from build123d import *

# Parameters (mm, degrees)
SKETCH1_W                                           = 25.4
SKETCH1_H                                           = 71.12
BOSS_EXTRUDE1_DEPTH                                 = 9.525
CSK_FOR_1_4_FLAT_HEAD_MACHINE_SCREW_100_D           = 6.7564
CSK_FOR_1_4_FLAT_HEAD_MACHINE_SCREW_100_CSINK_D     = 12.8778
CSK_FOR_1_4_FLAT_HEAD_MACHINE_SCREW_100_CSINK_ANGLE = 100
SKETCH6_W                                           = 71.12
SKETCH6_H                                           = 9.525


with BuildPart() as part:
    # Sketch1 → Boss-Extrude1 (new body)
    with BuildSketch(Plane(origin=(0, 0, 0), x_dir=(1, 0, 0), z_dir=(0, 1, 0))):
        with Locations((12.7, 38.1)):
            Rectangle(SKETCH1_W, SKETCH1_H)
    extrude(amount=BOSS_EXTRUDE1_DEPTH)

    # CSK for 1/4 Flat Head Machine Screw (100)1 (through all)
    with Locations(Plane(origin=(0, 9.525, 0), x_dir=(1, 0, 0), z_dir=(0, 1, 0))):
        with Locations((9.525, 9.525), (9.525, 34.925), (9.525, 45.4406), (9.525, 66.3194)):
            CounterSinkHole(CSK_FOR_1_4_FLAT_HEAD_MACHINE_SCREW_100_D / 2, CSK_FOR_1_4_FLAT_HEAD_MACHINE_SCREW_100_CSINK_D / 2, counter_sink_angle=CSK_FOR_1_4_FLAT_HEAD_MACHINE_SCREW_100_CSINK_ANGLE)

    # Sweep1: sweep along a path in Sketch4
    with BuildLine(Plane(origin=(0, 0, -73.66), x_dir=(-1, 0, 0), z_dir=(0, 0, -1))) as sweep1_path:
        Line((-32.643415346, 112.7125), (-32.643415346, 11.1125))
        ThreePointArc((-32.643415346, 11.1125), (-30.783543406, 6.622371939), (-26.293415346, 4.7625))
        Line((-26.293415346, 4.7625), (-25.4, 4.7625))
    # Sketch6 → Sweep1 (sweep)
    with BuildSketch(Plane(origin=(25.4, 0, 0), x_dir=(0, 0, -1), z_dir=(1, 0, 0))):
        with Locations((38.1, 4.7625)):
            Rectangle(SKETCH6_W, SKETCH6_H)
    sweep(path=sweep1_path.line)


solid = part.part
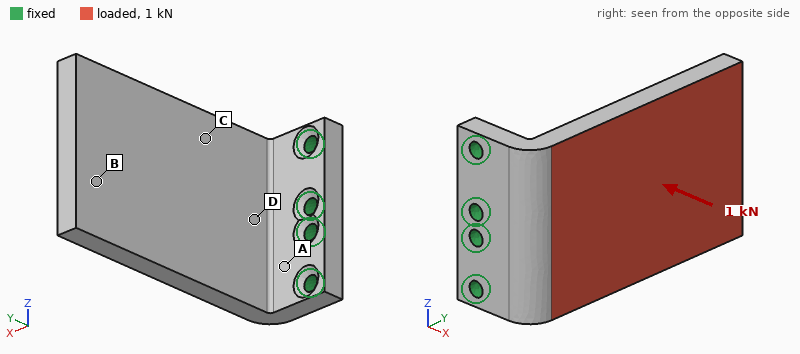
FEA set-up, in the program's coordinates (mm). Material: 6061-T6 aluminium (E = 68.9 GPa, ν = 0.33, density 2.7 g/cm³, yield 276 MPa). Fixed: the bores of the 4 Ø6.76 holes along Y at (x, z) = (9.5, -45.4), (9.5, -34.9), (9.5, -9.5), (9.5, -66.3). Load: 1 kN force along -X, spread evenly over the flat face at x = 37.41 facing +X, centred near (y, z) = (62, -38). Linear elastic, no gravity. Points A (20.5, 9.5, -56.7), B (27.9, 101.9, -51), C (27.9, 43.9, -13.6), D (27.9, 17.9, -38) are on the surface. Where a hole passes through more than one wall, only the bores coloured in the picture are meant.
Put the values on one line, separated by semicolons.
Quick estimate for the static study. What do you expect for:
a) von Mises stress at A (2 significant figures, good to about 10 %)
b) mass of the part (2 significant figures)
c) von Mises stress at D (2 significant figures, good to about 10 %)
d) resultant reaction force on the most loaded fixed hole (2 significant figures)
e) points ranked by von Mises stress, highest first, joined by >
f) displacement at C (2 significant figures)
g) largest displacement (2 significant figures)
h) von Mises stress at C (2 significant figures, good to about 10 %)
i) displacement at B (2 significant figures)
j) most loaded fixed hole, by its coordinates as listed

50 MPa; 250 g; 37 MPa; 440 N; A > D > C > B; 0.23 mm; 0.83 mm; 21 MPa; 0.72 mm; (9.5, -34.9)
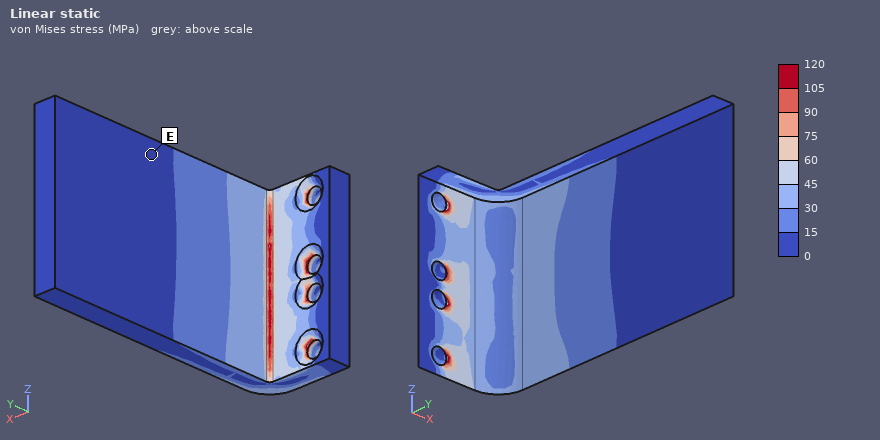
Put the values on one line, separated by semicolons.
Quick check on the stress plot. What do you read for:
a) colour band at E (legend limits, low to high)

0 to 15 MPa
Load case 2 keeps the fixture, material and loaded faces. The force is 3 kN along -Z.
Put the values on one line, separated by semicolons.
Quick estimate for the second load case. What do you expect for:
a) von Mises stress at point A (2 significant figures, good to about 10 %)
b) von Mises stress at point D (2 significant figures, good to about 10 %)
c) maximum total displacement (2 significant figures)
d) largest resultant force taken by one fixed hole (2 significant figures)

54 MPa; 25 MPa; 0.28 mm; 3.3 kN
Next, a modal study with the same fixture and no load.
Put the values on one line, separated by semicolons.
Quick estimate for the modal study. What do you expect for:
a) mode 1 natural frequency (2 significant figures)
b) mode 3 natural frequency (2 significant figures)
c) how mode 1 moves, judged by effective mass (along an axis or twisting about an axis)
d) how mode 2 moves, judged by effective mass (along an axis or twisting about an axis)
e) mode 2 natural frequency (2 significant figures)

500 Hz; 2200 Hz; along X; along Z; 1300 Hz
